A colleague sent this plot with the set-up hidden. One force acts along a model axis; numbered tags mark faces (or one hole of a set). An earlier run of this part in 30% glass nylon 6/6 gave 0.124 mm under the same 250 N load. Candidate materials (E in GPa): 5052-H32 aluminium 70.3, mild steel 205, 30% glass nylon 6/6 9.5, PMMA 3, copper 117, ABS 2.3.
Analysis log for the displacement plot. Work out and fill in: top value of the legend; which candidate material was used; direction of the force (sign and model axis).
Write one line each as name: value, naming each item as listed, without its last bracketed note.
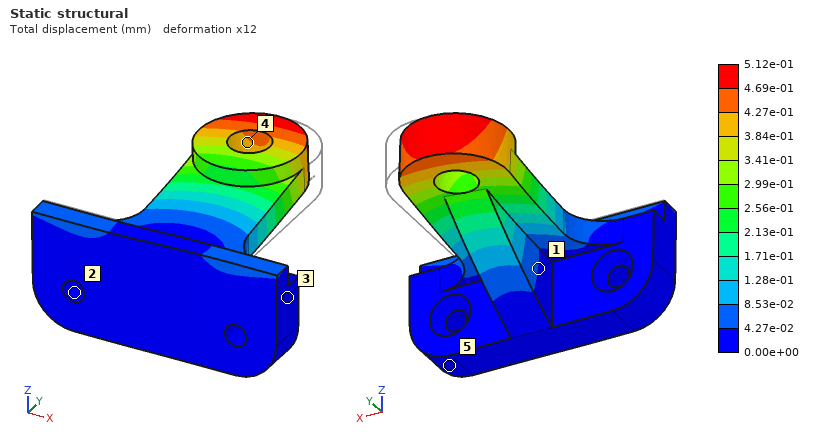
top value of the legend: 5.12e-01 mm
which candidate material was used: ABS
direction of the force: -X
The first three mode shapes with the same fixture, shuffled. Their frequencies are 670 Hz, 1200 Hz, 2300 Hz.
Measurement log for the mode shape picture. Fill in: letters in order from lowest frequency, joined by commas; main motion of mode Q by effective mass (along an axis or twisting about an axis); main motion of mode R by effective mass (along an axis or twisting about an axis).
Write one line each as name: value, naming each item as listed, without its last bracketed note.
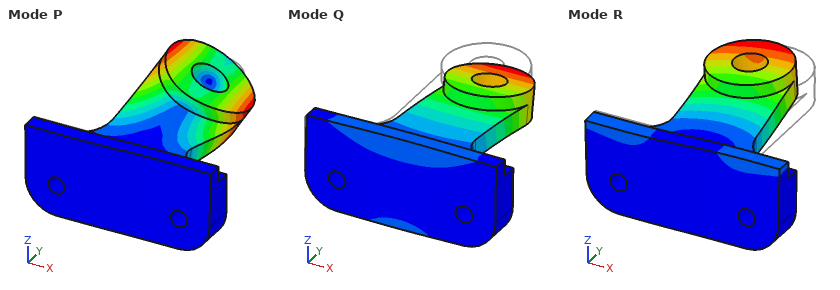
letters in order from lowest frequency, joined by commas: Q, R, P
main motion of mode Q by effective mass: along Z
main motion of mode R by effective mass: along X
